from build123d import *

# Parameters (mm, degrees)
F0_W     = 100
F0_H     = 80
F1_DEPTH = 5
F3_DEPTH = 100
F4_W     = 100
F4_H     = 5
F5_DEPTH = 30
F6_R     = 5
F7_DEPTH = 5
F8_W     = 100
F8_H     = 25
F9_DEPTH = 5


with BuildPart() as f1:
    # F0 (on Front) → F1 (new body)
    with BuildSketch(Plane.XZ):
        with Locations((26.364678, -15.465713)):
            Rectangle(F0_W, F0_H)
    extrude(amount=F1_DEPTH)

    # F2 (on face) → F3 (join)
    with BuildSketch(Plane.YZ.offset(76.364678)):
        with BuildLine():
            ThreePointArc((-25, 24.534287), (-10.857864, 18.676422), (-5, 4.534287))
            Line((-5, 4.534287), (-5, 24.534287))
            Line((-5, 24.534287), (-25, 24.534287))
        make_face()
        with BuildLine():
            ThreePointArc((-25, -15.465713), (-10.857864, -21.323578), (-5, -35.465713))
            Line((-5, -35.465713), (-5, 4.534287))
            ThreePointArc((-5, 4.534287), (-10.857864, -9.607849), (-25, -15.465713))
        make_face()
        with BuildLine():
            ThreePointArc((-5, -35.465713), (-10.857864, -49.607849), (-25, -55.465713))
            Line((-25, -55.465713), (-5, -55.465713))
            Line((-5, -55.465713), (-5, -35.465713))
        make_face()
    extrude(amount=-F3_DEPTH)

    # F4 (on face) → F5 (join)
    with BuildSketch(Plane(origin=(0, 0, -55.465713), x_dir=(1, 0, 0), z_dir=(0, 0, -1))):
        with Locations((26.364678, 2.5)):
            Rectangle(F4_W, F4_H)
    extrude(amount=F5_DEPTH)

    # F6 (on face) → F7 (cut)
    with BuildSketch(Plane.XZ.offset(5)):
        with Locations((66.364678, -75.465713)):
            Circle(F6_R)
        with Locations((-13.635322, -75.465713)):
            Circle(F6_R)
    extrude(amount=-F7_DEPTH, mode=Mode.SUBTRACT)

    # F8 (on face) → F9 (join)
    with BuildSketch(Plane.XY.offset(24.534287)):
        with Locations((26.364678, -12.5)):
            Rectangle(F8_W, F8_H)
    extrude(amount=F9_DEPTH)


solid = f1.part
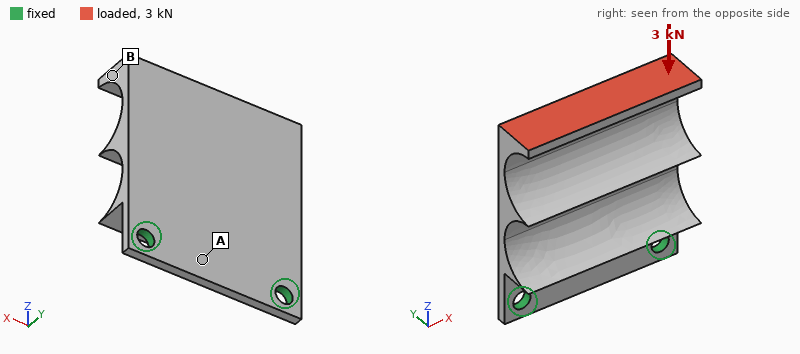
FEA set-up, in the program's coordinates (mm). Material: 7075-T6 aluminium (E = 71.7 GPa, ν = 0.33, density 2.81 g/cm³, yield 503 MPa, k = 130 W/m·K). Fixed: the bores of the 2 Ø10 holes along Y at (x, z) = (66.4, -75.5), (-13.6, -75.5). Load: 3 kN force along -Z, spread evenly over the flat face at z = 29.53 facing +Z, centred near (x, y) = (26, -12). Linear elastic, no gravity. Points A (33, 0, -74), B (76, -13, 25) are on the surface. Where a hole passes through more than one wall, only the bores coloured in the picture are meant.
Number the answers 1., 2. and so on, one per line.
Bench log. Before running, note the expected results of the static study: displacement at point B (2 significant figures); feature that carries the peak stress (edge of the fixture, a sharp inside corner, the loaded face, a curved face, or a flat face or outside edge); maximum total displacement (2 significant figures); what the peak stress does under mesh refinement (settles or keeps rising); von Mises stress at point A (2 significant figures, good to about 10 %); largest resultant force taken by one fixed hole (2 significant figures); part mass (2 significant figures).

1. 1.3 mm
2. edge of the fixture
3. 1.5 mm
4. keeps rising
5. 24 MPa
6. 1.5 kN
7. 280 g
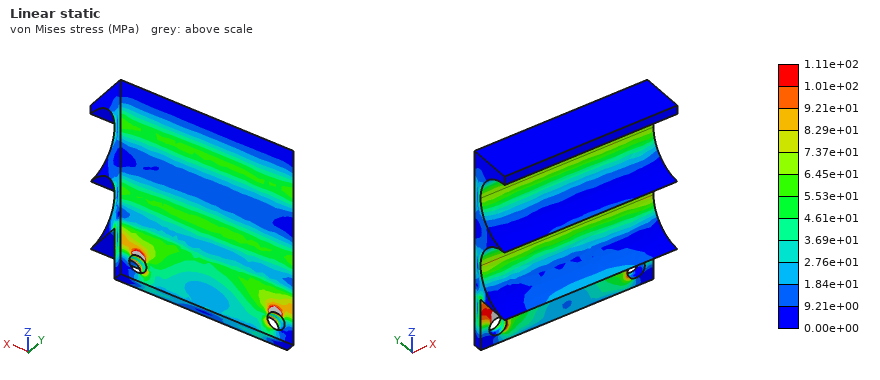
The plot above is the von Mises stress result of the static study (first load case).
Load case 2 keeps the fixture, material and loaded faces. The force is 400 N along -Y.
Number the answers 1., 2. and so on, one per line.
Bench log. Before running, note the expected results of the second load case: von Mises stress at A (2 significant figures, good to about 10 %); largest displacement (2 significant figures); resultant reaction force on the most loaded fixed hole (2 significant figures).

1. 30 MPa
2. 1.6 mm
3. 240 N
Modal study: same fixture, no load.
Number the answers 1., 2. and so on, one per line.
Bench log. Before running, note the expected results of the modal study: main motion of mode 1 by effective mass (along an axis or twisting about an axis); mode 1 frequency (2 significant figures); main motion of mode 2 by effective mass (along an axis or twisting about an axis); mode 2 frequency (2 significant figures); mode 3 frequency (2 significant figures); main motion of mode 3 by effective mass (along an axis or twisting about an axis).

1. along Y
2. 260 Hz
3. twisting about Z
4. 1100 Hz
5. 2000 Hz
6. along Y
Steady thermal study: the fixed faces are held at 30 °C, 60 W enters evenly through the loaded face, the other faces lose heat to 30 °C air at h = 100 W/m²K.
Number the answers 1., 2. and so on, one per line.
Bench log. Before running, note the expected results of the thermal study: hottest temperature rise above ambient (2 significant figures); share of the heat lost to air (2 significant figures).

1. 36 K
2. 77 %
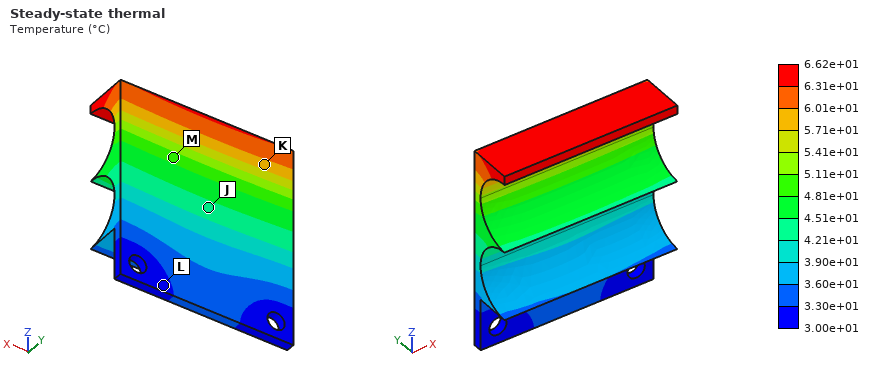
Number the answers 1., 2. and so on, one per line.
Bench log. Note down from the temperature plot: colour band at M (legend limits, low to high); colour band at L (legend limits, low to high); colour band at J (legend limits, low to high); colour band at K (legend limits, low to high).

1. 4.81e+01 to 5.11e+01 °C
2. 3.00e+01 to 3.30e+01 °C
3. 4.21e+01 to 4.51e+01 °C
4. 5.71e+01 to 6.01e+01 °C
